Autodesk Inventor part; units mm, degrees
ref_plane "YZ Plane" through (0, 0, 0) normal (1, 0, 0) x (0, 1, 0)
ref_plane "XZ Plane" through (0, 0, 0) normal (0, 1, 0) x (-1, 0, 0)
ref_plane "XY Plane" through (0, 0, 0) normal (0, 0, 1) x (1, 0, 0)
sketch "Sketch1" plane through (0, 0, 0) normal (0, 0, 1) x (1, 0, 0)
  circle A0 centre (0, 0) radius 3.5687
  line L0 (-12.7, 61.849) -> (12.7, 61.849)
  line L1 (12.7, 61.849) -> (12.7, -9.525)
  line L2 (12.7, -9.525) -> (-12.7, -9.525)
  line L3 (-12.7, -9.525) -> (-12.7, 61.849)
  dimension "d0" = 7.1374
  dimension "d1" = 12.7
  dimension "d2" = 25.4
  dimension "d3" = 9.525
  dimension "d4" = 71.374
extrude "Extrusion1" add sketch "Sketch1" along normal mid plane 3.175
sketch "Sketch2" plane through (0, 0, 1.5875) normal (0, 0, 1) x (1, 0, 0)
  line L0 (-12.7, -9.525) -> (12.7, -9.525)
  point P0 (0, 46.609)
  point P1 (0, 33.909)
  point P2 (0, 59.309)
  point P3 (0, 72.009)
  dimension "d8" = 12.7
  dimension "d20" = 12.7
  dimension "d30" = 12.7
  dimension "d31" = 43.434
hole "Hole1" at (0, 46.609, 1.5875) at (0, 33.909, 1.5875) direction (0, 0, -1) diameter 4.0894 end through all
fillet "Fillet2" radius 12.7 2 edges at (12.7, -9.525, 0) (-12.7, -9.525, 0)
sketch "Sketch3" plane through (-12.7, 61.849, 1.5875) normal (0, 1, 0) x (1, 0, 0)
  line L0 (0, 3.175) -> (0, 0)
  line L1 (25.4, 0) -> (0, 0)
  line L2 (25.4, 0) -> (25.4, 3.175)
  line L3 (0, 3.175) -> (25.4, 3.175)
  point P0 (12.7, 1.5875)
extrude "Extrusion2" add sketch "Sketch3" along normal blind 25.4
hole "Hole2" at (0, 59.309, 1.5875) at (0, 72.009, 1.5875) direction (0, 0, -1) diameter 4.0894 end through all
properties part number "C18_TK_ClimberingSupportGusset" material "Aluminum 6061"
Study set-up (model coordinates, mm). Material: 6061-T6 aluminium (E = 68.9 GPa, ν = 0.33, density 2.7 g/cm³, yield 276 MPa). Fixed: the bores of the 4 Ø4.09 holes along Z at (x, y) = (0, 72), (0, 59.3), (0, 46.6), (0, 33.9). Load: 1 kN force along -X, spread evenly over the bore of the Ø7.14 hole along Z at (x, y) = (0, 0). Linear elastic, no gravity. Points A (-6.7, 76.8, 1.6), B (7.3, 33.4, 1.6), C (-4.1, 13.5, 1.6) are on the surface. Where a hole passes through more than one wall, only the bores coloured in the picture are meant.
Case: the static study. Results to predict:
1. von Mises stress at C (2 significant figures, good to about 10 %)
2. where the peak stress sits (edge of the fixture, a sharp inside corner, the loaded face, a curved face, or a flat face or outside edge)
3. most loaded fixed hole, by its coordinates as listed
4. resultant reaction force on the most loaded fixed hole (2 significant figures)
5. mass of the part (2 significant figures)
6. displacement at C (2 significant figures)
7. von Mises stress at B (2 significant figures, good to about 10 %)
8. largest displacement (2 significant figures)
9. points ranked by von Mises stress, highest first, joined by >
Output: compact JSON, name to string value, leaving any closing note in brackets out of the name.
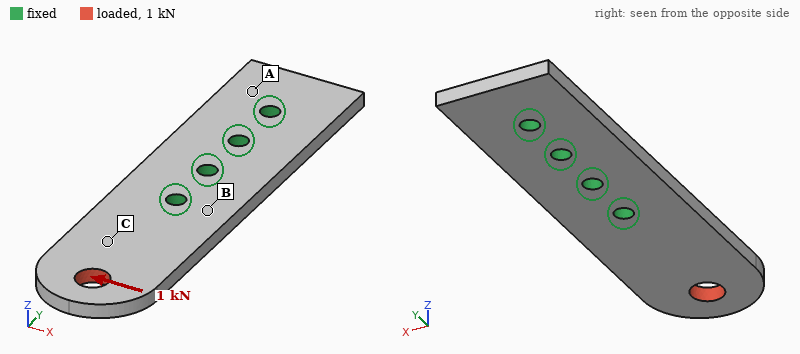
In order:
{"von Mises stress at C": "31 MPa", "where the peak stress sits": "edge of the fixture", "most loaded fixed hole, by its coordinates as listed": "(0, 33.9)", "resultant reaction force on the most loaded fixed hole": "2.3 kN", "mass of the part": "20 g", "displacement at C": "0.059 mm", "von Mises stress at B": "57 MPa", "largest displacement": "0.14 mm", "points ranked by von Mises stress, highest first, joined by >": "B > C > A"}
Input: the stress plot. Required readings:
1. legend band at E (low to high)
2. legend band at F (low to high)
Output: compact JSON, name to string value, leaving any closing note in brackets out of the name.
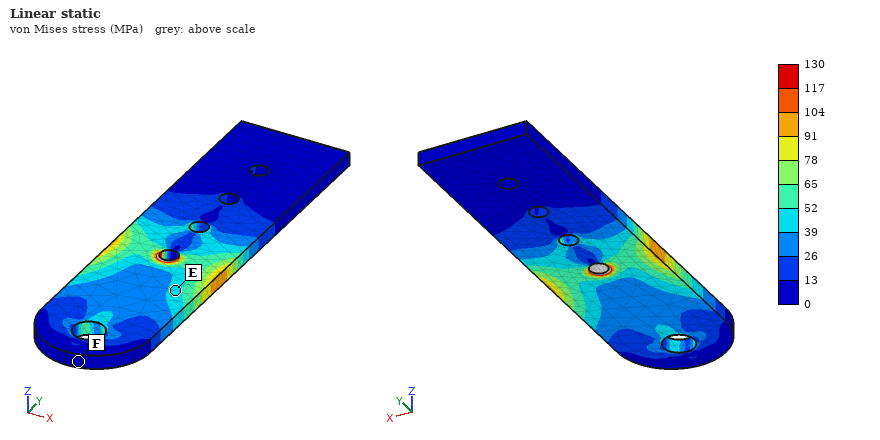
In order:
{"legend band at E": "39 to 52 MPa", "legend band at F": "0 to 13 MPa"}
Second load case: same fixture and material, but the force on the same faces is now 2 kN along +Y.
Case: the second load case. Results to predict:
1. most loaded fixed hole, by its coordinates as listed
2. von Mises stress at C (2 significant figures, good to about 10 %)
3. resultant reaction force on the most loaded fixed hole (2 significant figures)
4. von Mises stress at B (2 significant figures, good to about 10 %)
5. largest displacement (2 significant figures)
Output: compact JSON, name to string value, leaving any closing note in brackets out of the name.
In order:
{"most loaded fixed hole, by its coordinates as listed": "(0, 33.9)", "von Mises stress at C": "28 MPa", "resultant reaction force on the most loaded fixed hole": "1.4 kN", "von Mises stress at B": "16 MPa", "largest displacement": "20 µm"}
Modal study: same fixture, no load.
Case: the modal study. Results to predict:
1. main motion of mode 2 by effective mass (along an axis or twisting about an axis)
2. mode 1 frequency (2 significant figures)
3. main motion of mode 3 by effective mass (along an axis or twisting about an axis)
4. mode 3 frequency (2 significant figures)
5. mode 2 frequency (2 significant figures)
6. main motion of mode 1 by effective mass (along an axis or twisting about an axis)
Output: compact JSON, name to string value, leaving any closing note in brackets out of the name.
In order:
{"main motion of mode 2 by effective mass": "twisting about Y", "mode 1 frequency": "1600 Hz", "main motion of mode 3 by effective mass": "along X", "mode 3 frequency": "7600 Hz", "mode 2 frequency": "4900 Hz", "main motion of mode 1 by effective mass": "along Z"}
